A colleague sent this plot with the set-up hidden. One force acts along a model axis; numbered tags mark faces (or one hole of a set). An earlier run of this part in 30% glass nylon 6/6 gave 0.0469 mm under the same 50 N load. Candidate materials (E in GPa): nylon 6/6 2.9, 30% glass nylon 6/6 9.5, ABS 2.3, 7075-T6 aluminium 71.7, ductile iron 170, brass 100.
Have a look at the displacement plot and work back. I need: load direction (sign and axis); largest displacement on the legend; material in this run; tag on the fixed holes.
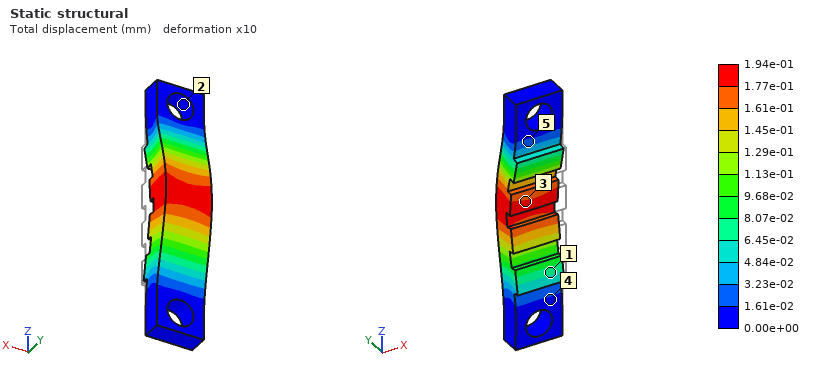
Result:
+Y
1.94e-01 mm
ABS
2
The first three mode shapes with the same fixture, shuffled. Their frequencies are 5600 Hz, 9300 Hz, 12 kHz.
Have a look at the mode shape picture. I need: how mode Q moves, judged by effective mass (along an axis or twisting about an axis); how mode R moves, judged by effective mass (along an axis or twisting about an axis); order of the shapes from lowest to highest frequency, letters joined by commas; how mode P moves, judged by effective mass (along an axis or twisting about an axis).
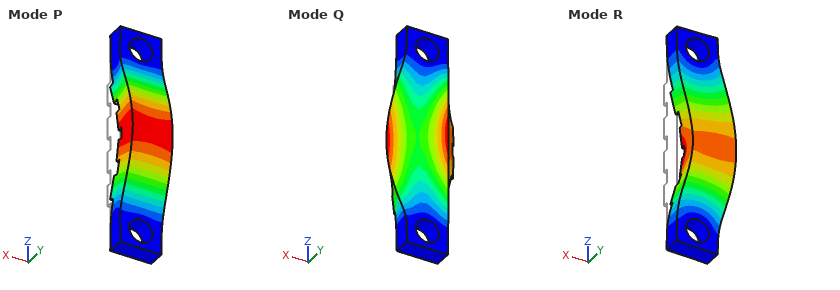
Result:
twisting about Z
along X
P, R, Q
along Y
